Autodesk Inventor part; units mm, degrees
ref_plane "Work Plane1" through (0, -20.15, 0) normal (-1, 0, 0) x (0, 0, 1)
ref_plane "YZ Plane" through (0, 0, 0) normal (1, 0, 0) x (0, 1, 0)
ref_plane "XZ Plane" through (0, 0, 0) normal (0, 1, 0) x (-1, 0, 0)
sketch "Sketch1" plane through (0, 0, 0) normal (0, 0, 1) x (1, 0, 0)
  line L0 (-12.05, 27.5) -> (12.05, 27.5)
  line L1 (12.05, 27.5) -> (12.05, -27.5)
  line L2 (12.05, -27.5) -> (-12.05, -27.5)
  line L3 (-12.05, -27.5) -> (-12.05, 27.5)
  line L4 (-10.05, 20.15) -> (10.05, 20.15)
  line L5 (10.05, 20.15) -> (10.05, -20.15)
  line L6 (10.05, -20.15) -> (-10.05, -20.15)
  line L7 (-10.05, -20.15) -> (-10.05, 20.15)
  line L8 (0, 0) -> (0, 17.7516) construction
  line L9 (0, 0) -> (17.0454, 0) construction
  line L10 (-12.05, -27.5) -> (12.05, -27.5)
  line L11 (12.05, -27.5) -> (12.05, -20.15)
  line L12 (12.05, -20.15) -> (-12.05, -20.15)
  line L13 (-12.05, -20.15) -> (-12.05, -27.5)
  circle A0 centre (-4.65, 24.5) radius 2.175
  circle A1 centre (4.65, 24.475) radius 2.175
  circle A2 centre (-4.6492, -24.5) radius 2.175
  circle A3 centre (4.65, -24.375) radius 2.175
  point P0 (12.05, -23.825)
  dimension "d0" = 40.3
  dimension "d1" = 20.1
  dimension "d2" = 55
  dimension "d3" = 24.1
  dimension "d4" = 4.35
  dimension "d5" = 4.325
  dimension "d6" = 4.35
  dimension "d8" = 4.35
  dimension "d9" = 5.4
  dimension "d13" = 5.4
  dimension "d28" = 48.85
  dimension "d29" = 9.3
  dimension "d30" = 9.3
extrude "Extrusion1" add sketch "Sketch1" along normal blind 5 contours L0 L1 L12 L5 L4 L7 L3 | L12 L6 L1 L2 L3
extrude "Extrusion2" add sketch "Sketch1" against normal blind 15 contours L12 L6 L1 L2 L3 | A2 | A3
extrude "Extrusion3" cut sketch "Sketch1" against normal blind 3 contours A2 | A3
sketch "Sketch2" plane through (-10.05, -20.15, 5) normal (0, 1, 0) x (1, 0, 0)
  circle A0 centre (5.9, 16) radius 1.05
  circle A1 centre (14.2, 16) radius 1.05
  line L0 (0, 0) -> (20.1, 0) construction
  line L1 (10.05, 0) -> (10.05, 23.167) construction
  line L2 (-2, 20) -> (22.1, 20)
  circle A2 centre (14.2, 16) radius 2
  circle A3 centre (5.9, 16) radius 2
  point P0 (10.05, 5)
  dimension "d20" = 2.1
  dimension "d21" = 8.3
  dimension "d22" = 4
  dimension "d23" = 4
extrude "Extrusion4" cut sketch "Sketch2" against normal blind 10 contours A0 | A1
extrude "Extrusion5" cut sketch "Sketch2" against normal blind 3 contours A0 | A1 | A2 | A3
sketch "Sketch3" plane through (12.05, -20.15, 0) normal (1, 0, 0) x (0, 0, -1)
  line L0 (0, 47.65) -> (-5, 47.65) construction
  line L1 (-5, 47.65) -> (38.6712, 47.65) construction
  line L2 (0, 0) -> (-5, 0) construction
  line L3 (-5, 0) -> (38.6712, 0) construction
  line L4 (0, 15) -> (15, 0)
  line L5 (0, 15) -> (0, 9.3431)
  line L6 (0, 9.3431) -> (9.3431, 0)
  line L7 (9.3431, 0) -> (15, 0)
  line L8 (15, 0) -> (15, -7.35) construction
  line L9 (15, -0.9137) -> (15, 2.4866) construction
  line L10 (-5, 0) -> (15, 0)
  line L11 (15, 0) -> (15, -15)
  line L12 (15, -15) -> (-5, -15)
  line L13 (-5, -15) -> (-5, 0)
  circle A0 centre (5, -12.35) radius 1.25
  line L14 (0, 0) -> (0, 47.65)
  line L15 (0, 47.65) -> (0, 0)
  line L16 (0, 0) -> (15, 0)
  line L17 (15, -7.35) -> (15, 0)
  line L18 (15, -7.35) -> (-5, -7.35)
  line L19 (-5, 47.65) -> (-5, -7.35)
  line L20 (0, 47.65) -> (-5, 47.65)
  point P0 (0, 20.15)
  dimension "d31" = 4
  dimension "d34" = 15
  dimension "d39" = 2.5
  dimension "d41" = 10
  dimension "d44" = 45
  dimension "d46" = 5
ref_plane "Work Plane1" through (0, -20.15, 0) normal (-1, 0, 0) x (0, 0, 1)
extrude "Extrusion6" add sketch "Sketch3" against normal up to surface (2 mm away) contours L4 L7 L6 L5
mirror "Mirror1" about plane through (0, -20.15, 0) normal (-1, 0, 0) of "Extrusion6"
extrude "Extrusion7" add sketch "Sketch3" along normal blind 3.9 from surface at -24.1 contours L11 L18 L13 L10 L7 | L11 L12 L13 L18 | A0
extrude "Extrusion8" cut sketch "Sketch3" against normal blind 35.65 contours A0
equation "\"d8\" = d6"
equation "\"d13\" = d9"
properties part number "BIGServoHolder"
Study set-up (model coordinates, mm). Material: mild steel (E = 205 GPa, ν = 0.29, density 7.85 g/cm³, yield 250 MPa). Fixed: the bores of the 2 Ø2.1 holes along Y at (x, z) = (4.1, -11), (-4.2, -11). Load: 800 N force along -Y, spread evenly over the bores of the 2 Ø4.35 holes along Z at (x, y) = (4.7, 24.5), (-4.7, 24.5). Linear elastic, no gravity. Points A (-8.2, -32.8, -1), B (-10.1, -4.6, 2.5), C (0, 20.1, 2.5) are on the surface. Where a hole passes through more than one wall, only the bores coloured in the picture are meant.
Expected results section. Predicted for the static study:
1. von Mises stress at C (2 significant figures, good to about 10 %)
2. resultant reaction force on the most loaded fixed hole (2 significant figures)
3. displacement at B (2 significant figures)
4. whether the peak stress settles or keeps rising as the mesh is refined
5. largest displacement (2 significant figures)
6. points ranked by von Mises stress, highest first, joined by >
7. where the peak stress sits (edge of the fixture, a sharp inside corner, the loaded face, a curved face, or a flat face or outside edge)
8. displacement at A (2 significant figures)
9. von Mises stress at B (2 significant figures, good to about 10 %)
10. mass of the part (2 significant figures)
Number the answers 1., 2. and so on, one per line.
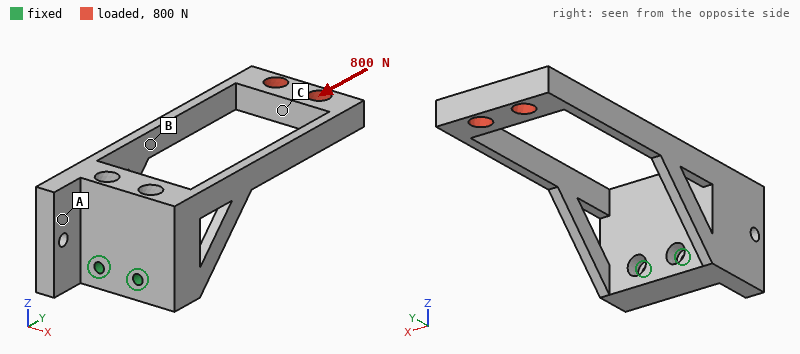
1. 73 MPa
2. 400 N
3. 30 µm
4. keeps rising
5. 75 µm
6. C > B > A
7. edge of the fixture
8. 13 µm
9. 38 MPa
10. 44 g
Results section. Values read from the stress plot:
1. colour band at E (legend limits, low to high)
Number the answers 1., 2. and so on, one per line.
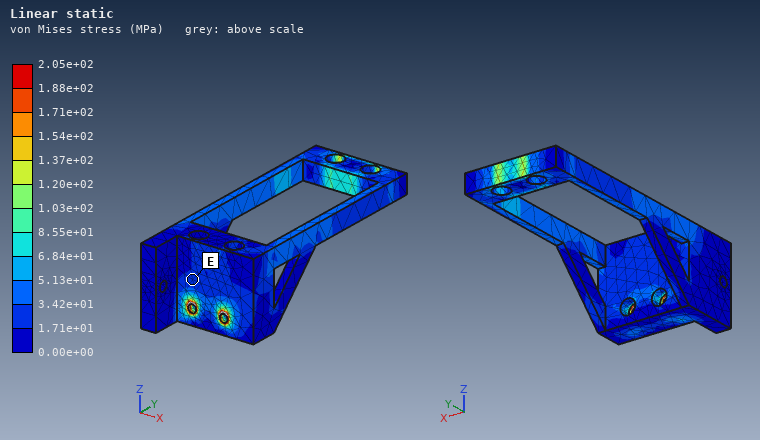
1. 1.71e+01 to 3.42e+01 MPa
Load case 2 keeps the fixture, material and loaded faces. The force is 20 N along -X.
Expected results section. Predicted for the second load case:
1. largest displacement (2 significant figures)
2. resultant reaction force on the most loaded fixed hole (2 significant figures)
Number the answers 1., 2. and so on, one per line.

1. 79 µm
2. 85 N
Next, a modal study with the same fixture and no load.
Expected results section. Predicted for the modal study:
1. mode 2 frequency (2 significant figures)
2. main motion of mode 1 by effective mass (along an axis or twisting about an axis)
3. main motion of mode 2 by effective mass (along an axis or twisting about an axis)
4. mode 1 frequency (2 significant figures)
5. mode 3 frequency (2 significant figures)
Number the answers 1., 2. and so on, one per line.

1. 1500 Hz
2. along X
3. along Z
4. 900 Hz
5. 3700 Hz
